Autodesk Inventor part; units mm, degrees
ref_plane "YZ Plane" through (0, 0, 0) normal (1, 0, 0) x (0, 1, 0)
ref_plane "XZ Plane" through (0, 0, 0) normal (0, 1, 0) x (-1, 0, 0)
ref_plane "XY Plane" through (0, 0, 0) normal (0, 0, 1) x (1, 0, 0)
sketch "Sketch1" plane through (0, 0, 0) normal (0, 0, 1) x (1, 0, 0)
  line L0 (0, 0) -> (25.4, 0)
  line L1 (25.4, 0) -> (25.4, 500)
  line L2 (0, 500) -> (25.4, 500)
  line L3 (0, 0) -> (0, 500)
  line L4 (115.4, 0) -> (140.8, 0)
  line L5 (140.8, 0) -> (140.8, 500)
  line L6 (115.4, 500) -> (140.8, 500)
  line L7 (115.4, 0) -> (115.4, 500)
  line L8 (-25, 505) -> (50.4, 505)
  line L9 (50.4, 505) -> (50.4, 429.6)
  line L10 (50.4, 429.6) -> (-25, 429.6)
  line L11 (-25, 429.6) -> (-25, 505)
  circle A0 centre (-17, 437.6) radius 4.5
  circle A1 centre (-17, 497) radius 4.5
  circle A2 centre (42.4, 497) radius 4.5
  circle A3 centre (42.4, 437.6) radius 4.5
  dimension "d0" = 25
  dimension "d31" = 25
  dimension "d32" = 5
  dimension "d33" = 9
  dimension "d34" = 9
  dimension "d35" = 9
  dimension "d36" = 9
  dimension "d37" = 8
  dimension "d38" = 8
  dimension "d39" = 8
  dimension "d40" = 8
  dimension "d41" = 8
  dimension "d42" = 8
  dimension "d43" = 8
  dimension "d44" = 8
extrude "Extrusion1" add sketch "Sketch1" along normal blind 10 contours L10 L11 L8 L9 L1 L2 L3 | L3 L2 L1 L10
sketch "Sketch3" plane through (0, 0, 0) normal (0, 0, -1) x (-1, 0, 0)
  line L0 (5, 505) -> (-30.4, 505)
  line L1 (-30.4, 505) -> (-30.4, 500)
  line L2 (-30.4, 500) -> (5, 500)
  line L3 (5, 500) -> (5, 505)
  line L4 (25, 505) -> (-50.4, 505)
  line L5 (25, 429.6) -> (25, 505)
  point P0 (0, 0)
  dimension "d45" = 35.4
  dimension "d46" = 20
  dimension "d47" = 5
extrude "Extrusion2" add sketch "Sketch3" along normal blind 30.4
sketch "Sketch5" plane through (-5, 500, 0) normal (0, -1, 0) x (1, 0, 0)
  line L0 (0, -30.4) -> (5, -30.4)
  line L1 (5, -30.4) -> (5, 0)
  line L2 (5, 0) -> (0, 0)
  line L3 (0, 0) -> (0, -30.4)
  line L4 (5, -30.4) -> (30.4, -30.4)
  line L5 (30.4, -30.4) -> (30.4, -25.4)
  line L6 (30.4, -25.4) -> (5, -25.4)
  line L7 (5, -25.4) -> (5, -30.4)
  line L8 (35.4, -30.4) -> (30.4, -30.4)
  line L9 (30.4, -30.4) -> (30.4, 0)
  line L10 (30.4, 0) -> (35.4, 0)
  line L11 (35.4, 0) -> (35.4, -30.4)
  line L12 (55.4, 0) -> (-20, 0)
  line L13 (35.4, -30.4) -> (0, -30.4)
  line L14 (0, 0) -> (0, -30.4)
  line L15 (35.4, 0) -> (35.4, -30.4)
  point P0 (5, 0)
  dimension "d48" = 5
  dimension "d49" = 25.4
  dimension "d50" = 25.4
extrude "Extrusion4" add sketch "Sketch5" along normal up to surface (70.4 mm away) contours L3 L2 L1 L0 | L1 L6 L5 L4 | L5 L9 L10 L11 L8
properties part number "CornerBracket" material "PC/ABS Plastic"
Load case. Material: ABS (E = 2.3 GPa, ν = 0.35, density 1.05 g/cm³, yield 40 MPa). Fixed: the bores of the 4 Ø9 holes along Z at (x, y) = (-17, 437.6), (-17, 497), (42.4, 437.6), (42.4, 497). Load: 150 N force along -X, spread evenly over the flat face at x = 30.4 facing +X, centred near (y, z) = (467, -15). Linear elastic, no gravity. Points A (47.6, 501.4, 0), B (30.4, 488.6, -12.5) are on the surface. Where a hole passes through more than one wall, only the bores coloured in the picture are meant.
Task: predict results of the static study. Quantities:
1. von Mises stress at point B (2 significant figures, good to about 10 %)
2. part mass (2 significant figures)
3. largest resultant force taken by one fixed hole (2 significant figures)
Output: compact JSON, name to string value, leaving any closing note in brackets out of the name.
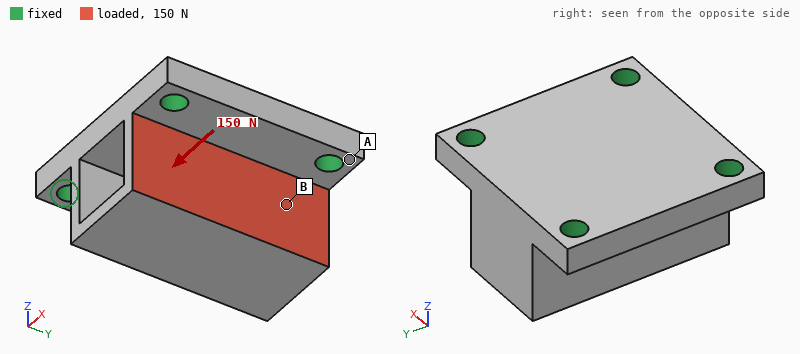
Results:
{"von Mises stress at point B": "0.41 MPa", "part mass": "95 g", "largest resultant force taken by one fixed hole": "67 N"}
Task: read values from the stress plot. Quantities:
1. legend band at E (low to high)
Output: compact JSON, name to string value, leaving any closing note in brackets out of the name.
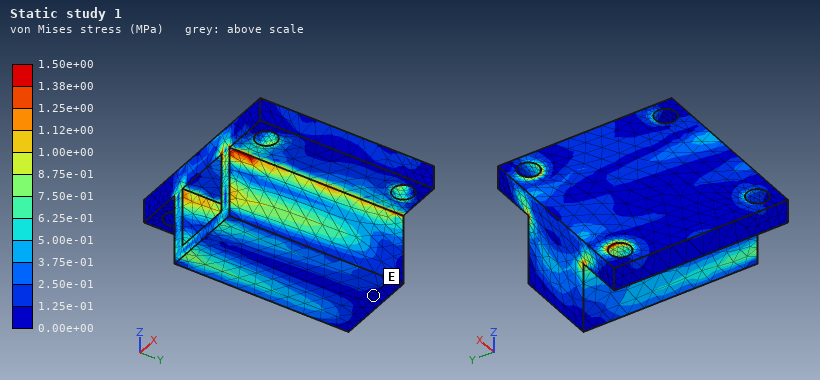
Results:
{"legend band at E": "0.00e+00 to 1.25e-01 MPa"}
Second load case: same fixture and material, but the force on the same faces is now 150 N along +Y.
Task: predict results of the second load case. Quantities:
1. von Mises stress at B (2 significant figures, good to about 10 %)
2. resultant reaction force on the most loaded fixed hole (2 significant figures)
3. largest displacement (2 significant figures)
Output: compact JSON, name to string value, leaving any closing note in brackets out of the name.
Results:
{"von Mises stress at B": "0.48 MPa", "resultant reaction force on the most loaded fixed hole": "65 N", "largest displacement": "29 µm"}
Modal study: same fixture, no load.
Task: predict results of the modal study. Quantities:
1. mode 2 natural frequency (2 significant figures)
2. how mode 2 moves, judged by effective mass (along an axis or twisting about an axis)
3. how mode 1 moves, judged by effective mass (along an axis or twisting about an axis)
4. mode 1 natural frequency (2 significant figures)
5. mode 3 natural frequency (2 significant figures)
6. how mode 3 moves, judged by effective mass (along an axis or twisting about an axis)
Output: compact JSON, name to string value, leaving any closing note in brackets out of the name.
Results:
{"mode 2 natural frequency": "2600 Hz", "how mode 2 moves, judged by effective mass": "along Y", "how mode 1 moves, judged by effective mass": "along X", "mode 1 natural frequency": "1500 Hz", "mode 3 natural frequency": "2700 Hz", "how mode 3 moves, judged by effective mass": "along Z"}
